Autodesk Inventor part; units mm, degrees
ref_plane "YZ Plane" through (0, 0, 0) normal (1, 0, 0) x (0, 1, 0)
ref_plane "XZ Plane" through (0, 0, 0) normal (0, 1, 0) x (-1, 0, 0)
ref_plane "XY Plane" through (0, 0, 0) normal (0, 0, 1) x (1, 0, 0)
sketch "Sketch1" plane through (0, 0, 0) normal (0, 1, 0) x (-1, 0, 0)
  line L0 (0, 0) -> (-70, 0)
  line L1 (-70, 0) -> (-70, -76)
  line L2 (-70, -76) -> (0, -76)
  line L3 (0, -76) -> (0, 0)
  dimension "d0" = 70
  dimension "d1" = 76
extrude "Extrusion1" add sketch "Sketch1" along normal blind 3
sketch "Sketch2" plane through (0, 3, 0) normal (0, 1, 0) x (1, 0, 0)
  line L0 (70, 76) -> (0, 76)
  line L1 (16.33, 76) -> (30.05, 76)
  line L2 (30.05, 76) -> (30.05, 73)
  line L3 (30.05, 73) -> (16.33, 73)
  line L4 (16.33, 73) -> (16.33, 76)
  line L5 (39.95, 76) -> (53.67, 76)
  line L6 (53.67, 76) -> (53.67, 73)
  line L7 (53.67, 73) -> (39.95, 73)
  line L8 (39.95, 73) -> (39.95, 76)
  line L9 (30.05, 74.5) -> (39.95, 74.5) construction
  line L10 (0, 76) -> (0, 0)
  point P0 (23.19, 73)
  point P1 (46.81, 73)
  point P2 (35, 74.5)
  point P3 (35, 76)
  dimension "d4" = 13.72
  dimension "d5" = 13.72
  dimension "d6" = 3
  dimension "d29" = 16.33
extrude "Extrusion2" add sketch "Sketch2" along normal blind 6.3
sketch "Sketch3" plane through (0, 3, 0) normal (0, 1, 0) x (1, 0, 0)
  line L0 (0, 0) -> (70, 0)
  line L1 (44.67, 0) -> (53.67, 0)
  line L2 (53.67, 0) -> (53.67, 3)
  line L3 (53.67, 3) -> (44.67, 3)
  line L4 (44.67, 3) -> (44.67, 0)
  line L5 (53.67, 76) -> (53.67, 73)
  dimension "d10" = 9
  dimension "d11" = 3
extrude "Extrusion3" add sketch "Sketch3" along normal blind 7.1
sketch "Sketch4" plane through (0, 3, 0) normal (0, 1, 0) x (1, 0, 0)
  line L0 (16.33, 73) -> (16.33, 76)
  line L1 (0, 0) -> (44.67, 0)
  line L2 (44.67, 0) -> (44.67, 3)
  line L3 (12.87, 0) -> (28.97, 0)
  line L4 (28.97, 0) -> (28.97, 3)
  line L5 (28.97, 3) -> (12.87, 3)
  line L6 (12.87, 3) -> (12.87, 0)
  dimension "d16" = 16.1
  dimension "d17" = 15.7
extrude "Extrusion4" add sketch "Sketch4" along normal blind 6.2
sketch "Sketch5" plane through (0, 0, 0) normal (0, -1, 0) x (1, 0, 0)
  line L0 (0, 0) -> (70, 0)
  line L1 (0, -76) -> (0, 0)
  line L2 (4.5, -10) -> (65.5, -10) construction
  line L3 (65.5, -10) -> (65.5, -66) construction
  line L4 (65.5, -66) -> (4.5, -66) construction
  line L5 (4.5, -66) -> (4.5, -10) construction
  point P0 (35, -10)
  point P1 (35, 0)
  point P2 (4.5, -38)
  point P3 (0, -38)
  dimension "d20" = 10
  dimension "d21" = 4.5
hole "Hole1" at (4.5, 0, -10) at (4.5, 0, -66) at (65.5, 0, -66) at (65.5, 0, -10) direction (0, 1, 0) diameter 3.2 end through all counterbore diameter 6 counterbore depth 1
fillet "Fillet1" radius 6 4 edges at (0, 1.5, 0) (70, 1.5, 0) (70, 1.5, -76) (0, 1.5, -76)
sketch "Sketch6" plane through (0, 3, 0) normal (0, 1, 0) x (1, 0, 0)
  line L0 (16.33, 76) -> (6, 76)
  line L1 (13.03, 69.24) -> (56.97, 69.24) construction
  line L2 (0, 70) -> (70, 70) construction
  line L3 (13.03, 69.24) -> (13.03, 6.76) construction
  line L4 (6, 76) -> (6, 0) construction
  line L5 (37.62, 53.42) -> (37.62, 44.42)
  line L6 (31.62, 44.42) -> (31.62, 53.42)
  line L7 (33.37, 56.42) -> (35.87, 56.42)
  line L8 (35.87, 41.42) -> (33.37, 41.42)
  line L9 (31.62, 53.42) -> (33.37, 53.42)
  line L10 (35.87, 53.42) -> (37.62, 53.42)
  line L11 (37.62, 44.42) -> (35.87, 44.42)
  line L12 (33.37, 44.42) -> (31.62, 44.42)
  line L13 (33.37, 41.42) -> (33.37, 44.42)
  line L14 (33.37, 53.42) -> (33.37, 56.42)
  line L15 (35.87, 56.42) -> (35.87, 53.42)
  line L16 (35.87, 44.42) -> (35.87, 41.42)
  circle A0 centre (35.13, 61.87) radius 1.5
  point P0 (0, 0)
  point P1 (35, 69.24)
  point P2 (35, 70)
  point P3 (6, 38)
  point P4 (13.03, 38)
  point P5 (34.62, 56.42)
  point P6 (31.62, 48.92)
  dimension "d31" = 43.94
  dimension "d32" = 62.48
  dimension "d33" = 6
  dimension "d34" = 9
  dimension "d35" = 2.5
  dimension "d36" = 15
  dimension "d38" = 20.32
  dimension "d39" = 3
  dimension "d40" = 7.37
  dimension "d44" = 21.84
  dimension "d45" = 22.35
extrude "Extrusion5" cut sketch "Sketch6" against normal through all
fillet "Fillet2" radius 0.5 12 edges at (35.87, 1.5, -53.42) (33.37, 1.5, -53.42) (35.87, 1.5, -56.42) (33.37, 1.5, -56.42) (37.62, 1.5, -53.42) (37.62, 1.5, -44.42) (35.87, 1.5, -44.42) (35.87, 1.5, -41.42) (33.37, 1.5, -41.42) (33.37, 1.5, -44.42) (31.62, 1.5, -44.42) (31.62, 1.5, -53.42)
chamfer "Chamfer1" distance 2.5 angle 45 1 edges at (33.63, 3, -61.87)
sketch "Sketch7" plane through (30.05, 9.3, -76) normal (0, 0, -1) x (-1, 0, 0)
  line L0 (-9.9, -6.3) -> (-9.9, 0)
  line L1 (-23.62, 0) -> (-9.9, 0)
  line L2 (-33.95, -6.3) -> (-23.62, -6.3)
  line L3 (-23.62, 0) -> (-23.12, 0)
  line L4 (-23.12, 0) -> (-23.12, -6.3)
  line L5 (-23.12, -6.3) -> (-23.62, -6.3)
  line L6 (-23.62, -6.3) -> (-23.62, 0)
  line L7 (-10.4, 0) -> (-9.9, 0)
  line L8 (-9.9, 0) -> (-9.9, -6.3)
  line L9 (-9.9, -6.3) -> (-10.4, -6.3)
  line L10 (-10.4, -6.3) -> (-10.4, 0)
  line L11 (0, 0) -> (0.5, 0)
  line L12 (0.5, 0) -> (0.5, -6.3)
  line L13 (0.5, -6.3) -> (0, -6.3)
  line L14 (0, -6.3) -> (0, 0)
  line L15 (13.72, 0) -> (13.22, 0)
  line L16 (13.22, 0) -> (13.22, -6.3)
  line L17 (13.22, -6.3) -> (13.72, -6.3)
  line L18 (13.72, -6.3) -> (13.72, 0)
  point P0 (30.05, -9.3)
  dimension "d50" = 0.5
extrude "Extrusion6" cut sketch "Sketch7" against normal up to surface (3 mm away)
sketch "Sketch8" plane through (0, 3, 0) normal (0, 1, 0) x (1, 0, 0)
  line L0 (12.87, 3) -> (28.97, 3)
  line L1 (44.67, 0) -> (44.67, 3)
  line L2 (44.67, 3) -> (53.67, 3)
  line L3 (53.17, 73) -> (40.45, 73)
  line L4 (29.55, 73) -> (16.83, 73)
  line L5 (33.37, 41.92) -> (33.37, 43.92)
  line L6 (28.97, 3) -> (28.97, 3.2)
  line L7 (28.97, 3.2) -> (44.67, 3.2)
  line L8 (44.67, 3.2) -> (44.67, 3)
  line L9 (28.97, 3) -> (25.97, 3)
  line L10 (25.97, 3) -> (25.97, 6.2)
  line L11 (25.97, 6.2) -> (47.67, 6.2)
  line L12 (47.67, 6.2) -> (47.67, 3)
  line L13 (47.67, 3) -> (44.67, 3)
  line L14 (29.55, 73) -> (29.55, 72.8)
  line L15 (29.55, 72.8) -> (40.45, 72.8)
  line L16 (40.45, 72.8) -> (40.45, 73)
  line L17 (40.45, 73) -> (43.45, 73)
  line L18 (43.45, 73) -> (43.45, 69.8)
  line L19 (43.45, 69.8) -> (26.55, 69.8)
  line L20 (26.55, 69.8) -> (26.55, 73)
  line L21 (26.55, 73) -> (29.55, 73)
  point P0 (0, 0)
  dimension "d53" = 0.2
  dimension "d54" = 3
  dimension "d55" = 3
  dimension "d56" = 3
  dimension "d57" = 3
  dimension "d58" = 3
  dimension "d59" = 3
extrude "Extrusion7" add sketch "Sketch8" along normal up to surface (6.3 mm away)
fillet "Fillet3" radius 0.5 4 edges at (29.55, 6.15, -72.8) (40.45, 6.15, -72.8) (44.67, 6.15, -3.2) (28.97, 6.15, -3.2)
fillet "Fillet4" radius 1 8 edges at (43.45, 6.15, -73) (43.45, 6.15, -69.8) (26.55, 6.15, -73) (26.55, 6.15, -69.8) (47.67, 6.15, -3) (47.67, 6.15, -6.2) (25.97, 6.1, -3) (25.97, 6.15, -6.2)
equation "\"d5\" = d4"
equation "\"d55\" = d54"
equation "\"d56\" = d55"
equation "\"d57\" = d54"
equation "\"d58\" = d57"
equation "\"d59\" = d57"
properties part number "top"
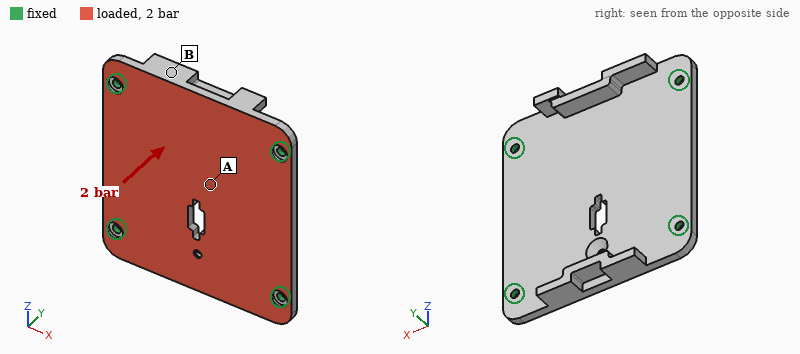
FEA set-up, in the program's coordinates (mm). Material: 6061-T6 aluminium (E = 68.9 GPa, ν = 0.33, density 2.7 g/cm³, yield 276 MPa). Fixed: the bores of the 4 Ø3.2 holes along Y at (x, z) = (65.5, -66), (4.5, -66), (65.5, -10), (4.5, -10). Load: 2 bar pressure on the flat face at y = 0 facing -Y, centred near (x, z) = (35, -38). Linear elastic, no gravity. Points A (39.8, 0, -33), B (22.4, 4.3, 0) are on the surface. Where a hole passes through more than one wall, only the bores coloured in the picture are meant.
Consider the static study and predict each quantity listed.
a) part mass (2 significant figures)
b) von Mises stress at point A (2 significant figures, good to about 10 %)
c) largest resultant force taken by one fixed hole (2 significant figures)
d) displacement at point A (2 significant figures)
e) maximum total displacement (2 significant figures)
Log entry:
46 g
27 MPa
310 N
0.11 mm
0.12 mm
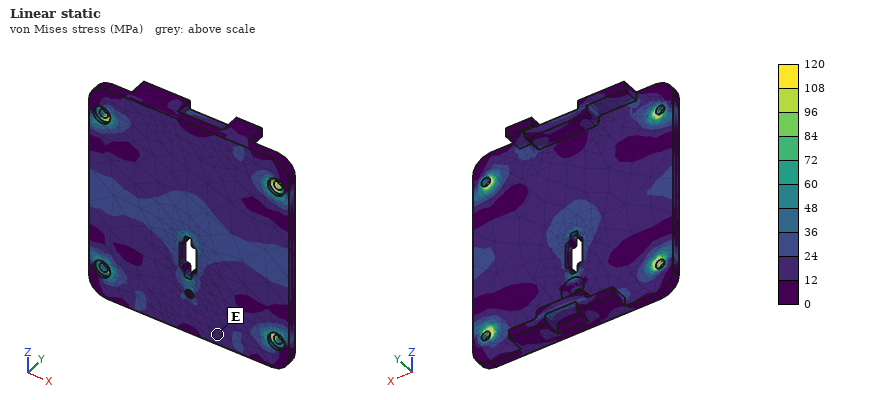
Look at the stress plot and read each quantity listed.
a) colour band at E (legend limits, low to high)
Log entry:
12 to 24 MPa
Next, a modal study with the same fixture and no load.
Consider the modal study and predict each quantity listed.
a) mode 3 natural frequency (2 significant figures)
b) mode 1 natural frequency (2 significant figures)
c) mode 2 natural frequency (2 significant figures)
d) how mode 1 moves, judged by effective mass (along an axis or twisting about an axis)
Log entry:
4400 Hz
2800 Hz
4300 Hz
along Y
